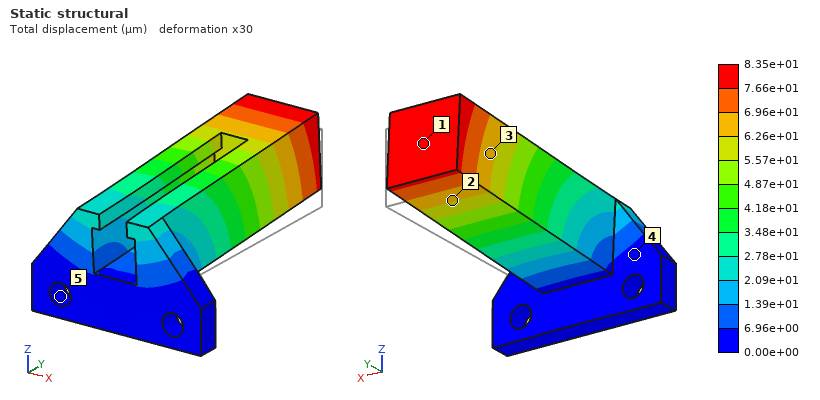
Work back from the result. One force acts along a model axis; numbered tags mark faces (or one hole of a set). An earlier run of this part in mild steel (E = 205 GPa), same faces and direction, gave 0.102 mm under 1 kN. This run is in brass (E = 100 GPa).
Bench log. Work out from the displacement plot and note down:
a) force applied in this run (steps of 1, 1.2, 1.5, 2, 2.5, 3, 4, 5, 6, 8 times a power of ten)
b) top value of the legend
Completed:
400 N
8.35e+01 µm
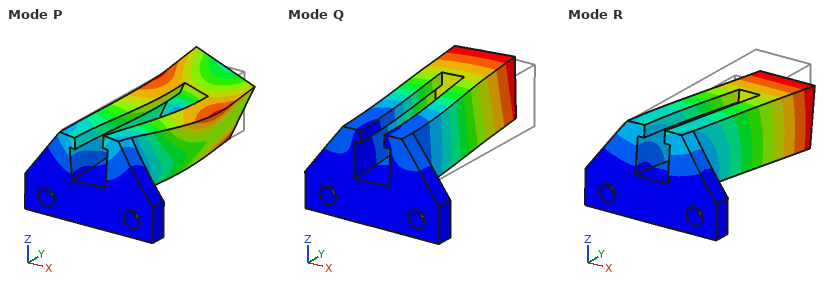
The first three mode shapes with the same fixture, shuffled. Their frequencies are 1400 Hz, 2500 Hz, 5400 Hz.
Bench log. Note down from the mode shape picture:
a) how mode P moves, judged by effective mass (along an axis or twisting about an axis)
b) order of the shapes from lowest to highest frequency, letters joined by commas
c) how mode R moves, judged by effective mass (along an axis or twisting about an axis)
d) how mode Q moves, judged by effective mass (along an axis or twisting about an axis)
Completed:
twisting about Y
R, Q, P
along Z
along X
